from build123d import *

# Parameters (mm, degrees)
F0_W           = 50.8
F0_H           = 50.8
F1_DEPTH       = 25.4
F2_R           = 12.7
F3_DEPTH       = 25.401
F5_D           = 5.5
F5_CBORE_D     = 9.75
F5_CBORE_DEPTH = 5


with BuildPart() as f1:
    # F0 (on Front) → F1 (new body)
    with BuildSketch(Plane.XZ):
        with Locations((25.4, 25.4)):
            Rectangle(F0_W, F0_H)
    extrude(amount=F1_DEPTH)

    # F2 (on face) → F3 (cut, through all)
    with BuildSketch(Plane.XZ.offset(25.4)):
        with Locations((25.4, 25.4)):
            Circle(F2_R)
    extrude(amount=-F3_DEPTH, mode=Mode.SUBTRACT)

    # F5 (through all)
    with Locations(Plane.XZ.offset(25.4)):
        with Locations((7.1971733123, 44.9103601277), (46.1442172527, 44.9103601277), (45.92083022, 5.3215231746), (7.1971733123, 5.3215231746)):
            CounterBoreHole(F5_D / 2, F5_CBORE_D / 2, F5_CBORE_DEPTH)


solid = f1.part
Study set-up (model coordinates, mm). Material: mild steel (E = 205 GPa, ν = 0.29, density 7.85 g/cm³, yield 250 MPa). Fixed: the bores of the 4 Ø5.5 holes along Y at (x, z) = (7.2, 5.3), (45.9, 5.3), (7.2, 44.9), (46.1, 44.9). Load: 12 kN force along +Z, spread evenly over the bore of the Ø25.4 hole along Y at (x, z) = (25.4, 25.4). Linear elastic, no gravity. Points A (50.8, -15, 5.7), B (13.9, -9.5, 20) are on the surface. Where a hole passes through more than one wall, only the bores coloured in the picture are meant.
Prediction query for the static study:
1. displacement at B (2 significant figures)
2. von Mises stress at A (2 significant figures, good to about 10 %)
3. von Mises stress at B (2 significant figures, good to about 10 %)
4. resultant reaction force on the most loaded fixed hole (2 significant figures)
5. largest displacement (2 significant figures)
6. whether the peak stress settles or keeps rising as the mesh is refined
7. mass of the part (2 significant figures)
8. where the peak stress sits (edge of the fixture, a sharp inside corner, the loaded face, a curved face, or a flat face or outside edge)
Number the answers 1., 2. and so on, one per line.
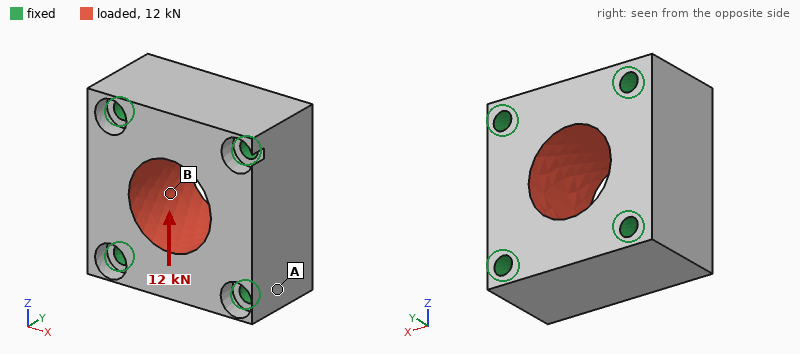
1. 0.74 µm
2. 4.8 MPa
3. 12 MPa
4. 3.3 kN
5. 1.7 µm
6. keeps rising
7. 390 g
8. edge of the fixture
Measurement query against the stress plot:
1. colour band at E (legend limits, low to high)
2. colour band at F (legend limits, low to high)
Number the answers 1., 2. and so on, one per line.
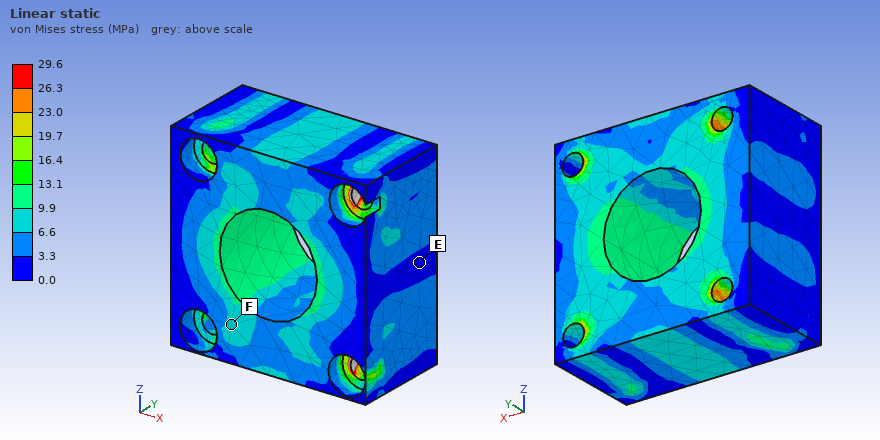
1. 0.0 to 3.3 MPa
2. 6.6 to 9.9 MPa
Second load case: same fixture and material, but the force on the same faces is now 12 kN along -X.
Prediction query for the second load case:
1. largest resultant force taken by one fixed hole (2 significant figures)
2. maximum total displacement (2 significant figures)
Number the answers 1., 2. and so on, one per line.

1. 3.3 kN
2. 1.7 µm
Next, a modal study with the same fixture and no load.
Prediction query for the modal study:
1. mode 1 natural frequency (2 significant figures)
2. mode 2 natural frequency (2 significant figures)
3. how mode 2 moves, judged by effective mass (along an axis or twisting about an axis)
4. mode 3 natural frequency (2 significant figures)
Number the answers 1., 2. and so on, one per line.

1. 25 kHz
2. 30 kHz
3. along Y
4. 33 kHz
